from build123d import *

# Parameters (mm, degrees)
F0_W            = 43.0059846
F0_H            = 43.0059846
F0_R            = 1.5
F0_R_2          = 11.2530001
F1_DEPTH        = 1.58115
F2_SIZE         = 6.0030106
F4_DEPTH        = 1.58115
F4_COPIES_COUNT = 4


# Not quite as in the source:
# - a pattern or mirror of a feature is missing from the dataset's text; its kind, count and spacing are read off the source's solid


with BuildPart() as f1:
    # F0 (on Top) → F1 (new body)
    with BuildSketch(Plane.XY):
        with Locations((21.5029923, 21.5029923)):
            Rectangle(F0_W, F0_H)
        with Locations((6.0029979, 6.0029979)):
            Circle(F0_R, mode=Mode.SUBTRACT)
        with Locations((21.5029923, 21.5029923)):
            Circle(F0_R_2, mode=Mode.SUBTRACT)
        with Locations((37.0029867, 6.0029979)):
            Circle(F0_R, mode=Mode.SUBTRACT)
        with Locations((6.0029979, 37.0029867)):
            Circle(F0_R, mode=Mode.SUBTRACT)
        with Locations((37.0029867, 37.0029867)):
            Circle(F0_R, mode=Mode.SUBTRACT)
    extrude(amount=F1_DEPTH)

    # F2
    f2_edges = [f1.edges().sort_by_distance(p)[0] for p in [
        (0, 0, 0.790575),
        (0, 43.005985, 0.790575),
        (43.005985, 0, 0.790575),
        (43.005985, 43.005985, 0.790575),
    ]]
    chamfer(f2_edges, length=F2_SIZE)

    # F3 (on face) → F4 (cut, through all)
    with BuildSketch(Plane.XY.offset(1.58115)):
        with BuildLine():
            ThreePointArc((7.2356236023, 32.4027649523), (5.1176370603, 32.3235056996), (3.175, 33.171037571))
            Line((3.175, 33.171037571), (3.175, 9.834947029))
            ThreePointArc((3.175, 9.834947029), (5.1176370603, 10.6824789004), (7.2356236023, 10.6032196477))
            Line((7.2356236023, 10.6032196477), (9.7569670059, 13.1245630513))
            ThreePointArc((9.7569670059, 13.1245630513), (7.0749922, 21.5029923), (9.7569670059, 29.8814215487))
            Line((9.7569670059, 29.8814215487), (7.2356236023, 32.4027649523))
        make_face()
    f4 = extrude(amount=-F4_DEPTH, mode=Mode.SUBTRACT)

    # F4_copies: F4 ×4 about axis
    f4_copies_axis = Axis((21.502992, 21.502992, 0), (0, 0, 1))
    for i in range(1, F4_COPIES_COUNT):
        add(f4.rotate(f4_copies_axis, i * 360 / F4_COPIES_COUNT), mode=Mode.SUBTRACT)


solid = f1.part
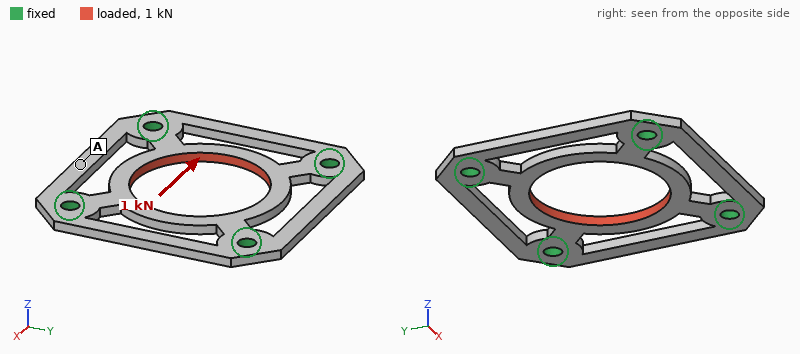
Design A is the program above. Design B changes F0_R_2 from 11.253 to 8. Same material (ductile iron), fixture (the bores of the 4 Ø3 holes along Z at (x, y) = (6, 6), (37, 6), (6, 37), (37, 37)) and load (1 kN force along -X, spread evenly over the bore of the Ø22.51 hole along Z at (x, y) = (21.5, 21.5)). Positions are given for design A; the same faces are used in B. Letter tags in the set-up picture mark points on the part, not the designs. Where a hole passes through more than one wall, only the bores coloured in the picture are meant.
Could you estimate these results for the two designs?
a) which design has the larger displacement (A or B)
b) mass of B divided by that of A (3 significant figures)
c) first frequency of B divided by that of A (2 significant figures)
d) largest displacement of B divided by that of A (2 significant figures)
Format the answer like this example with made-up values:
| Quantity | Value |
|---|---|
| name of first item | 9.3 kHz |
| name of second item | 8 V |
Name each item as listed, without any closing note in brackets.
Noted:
| Quantity | Value |
|---|---|
| which design has the larger displacement | A |
| mass of B divided by that of A | 1.21 |
| first frequency of B divided by that of A | 0.74 |
| largest displacement of B divided by that of A | 0.33 |
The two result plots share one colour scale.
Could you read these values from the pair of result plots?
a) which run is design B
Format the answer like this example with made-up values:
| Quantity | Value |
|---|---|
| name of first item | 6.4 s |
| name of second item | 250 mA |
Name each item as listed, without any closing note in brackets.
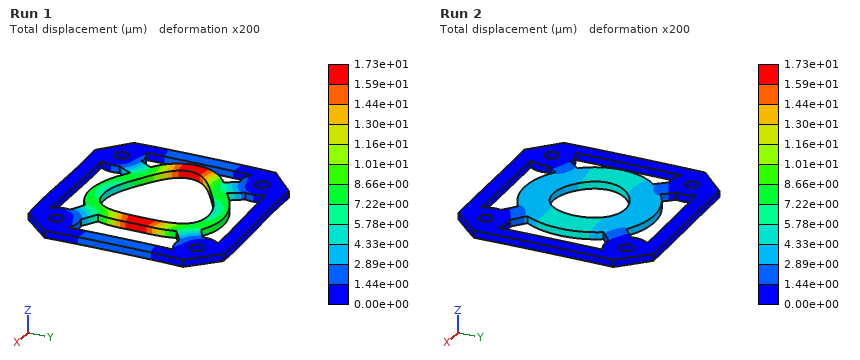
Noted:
| Quantity | Value |
|---|---|
| which run is design B | Run 2 |
